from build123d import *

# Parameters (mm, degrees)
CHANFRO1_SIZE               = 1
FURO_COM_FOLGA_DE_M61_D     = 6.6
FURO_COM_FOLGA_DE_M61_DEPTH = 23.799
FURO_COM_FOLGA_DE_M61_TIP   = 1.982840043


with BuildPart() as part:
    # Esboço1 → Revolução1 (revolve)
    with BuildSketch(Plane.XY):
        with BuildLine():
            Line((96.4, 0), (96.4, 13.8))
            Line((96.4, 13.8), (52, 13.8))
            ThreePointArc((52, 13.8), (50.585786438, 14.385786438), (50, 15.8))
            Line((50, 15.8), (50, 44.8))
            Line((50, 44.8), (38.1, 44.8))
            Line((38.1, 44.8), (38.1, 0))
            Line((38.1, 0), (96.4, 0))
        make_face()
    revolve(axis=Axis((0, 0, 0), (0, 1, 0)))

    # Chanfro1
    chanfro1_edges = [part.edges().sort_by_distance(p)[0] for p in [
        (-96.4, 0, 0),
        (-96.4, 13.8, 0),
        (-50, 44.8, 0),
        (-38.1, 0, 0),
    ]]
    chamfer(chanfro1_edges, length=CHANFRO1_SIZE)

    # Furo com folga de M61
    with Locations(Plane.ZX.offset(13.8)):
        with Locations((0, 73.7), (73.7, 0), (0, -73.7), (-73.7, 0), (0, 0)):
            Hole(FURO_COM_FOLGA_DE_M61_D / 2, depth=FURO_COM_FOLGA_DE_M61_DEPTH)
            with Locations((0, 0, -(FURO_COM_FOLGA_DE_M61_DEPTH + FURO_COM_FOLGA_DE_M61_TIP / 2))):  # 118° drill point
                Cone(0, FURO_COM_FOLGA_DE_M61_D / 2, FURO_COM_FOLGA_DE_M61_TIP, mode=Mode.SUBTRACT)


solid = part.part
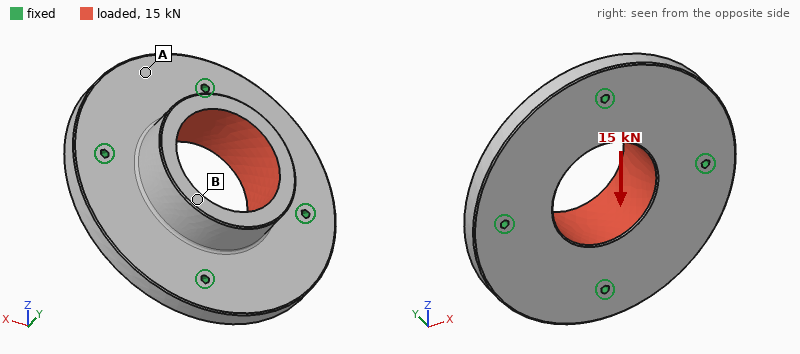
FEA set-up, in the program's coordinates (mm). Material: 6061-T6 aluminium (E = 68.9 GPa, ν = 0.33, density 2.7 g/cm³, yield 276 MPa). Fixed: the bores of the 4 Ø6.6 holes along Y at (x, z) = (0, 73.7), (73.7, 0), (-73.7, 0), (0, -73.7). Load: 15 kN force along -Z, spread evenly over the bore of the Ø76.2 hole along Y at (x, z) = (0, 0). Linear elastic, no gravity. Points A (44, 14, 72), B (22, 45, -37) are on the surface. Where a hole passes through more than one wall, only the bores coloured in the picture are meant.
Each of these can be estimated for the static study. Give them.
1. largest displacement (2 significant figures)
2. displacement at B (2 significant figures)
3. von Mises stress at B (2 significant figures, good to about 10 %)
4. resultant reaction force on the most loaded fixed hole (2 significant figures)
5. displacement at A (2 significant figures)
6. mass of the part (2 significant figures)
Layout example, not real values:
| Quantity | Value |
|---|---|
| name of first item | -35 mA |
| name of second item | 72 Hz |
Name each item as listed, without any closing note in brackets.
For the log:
| Quantity | Value |
|---|---|
| largest displacement | 17 µm |
| displacement at B | 17 µm |
| von Mises stress at B | 5.5 MPa |
| resultant reaction force on the most loaded fixed hole | 4.4 kN |
| displacement at A | 6.5 µm |
| mass of the part | 1.2 kg |
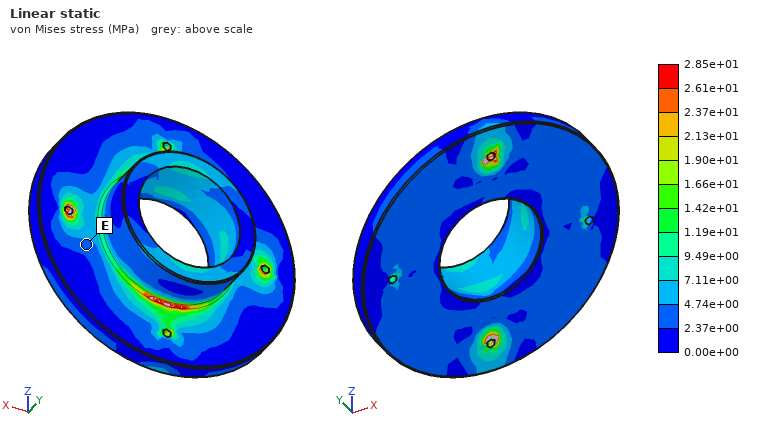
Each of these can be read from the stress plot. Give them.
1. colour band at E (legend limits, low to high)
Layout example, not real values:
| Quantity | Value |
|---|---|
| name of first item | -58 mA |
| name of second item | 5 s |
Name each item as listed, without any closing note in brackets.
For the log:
| Quantity | Value |
|---|---|
| colour band at E | 2.37e+00 to 4.74e+00 MPa |
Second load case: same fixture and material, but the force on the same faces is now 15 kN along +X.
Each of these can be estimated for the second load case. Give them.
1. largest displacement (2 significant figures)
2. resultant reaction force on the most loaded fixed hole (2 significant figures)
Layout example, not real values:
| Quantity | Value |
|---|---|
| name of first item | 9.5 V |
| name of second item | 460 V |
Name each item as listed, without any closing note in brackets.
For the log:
| Quantity | Value |
|---|---|
| largest displacement | 17 µm |
| resultant reaction force on the most loaded fixed hole | 4.4 kN |
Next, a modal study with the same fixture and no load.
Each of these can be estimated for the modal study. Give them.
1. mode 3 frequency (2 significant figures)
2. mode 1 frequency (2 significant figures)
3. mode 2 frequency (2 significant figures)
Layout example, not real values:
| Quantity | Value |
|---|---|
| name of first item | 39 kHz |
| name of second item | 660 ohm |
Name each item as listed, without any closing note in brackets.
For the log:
| Quantity | Value |
|---|---|
| mode 3 frequency | 4100 Hz |
| mode 1 frequency | 3700 Hz |
| mode 2 frequency | 4100 Hz |
